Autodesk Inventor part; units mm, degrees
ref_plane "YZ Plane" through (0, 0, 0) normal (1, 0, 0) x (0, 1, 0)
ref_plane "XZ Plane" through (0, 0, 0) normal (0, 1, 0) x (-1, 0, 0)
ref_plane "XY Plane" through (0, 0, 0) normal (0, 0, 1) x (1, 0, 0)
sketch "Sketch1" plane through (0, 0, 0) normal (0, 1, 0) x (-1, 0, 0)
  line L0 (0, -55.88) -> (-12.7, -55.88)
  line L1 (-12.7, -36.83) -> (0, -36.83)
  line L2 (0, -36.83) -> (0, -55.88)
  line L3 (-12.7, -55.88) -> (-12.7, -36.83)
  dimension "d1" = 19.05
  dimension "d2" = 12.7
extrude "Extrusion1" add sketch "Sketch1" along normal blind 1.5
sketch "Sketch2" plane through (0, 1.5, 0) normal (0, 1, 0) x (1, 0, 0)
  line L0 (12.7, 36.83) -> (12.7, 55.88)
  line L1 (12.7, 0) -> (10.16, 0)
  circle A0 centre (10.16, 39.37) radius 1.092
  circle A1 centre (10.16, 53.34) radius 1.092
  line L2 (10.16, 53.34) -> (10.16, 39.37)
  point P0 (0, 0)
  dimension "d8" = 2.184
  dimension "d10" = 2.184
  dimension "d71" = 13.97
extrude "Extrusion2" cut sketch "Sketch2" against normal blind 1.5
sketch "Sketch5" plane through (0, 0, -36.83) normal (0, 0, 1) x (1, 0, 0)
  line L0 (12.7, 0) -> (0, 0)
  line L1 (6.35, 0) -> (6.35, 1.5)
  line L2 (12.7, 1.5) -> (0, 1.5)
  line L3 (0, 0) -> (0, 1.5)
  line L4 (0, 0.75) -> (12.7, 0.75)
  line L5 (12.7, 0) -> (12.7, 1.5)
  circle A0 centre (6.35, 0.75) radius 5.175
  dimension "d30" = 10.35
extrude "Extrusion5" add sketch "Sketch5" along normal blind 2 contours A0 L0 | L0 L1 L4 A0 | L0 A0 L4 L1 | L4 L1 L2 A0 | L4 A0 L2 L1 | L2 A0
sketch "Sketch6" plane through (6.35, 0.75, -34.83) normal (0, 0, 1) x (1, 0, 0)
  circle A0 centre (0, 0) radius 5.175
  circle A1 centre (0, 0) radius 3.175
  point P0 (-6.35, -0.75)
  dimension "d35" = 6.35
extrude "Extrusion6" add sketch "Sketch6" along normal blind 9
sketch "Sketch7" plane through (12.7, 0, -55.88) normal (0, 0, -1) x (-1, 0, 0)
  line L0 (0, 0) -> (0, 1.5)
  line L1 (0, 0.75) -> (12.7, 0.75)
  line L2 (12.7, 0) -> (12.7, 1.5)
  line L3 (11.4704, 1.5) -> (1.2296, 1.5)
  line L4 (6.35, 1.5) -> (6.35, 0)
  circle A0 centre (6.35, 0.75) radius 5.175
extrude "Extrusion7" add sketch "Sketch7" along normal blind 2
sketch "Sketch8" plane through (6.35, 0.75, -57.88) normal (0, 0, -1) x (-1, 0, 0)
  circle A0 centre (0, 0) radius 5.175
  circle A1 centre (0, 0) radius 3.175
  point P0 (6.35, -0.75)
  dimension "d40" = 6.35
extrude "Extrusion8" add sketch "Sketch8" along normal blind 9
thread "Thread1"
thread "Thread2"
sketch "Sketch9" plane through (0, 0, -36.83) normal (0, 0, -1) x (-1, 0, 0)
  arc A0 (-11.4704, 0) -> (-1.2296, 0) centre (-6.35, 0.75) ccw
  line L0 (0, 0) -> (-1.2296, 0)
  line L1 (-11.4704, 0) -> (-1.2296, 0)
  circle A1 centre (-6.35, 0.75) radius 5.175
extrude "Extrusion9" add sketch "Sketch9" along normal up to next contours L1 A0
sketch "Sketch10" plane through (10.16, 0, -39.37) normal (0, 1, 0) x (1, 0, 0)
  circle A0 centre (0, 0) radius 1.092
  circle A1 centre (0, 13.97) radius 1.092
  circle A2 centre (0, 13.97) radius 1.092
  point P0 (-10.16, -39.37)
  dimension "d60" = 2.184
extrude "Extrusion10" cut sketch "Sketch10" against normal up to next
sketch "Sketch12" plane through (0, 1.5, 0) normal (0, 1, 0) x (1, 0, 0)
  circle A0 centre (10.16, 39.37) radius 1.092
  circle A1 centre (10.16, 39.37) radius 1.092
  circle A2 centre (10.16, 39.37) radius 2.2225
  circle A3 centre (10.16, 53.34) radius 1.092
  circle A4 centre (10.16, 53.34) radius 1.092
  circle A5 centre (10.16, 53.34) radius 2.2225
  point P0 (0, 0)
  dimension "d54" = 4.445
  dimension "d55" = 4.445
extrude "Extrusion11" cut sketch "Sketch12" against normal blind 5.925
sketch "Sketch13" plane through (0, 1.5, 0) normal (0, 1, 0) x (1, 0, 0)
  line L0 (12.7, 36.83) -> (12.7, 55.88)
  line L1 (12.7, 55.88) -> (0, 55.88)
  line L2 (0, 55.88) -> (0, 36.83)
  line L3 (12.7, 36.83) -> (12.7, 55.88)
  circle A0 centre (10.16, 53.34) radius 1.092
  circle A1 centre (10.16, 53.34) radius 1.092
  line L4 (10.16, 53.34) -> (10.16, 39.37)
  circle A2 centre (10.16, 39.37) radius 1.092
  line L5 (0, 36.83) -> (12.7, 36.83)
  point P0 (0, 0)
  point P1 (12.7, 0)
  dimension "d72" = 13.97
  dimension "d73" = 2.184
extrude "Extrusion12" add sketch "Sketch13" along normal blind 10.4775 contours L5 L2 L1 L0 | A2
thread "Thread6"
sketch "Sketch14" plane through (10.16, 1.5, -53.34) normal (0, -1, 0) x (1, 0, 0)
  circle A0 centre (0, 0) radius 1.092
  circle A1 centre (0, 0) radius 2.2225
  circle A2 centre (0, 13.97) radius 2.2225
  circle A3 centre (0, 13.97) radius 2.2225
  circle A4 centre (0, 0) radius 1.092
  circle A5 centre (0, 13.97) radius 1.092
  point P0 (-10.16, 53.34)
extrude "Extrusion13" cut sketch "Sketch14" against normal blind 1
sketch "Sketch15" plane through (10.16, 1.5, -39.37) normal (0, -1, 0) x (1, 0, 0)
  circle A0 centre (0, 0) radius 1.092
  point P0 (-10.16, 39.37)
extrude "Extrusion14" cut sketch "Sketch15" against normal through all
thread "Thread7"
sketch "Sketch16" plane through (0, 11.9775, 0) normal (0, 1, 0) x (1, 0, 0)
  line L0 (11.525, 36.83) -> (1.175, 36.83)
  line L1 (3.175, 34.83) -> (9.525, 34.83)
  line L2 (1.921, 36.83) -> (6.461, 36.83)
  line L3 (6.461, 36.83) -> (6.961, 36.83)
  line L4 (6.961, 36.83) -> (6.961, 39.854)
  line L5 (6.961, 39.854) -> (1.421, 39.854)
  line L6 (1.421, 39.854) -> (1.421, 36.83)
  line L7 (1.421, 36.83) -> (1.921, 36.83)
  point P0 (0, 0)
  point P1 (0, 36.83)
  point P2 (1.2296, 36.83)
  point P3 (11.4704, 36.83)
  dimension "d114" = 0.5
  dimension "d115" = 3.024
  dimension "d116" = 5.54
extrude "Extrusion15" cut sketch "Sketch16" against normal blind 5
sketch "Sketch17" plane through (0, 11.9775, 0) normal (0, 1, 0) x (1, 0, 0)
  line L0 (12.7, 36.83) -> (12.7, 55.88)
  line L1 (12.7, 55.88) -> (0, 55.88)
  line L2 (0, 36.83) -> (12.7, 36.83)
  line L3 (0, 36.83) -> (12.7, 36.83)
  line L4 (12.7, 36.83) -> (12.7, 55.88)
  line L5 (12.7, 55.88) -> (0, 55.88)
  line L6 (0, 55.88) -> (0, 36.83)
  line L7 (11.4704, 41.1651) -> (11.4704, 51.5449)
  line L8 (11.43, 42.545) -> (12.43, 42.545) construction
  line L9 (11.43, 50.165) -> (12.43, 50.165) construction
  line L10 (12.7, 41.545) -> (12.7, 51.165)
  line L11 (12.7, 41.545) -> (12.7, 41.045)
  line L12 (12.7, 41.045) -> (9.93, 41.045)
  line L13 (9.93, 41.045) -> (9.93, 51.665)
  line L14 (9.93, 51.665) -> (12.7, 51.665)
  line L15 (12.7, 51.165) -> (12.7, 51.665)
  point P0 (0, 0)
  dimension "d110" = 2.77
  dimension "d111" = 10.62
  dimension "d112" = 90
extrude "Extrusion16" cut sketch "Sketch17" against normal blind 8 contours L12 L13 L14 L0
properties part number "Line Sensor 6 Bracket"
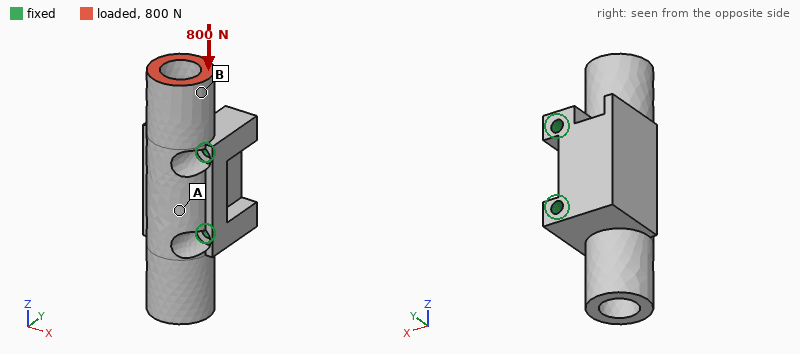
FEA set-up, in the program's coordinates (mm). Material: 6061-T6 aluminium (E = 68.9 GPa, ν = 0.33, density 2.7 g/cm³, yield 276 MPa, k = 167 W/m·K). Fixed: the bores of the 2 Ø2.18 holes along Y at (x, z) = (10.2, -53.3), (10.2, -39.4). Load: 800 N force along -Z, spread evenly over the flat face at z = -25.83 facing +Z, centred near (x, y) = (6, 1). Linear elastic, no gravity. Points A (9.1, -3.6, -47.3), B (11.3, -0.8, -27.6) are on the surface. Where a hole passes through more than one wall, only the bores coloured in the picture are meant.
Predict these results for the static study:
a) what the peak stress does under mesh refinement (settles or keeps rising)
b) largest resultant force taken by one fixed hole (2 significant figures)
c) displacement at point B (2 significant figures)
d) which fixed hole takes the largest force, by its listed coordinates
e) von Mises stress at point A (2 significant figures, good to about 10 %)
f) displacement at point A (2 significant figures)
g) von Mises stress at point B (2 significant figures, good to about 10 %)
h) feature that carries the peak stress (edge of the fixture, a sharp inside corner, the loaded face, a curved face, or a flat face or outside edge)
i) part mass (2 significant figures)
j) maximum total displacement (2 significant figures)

keeps rising
580 N
6.4 µm
(10.2, -39.4)
4.7 MPa
1.7 µm
16 MPa
edge of the fixture
12 g
8.2 µm
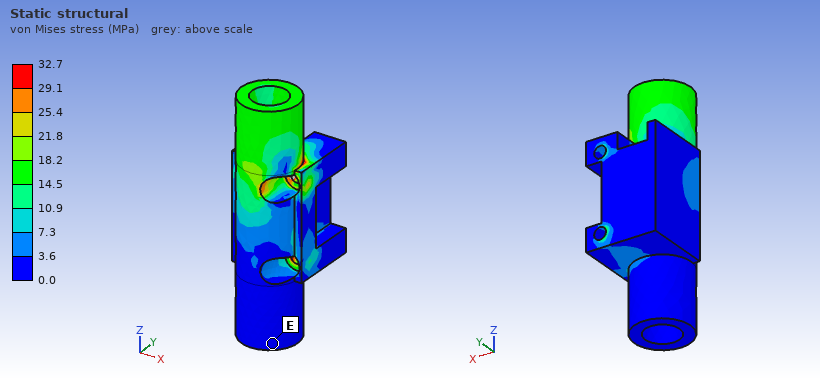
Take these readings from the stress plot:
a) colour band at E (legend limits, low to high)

0.0 to 3.6 MPa
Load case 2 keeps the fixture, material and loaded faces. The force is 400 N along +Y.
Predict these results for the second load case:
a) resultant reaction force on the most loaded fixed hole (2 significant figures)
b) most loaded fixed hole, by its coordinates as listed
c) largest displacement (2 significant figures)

670 N
(10.2, -39.4)
28 µm
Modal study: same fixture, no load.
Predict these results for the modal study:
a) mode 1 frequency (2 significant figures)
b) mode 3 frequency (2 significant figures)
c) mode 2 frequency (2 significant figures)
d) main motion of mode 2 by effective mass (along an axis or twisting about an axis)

21 kHz
24 kHz
22 kHz
twisting about X
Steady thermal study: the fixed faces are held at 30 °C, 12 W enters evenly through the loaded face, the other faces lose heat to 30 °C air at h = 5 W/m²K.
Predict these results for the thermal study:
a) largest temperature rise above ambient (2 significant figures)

20 K
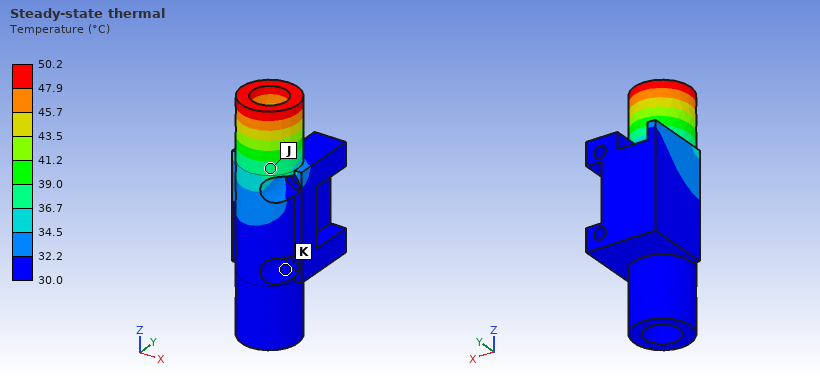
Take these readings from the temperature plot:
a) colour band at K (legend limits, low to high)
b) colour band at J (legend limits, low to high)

30.0 to 32.2 °C
36.7 to 39.0 °C
